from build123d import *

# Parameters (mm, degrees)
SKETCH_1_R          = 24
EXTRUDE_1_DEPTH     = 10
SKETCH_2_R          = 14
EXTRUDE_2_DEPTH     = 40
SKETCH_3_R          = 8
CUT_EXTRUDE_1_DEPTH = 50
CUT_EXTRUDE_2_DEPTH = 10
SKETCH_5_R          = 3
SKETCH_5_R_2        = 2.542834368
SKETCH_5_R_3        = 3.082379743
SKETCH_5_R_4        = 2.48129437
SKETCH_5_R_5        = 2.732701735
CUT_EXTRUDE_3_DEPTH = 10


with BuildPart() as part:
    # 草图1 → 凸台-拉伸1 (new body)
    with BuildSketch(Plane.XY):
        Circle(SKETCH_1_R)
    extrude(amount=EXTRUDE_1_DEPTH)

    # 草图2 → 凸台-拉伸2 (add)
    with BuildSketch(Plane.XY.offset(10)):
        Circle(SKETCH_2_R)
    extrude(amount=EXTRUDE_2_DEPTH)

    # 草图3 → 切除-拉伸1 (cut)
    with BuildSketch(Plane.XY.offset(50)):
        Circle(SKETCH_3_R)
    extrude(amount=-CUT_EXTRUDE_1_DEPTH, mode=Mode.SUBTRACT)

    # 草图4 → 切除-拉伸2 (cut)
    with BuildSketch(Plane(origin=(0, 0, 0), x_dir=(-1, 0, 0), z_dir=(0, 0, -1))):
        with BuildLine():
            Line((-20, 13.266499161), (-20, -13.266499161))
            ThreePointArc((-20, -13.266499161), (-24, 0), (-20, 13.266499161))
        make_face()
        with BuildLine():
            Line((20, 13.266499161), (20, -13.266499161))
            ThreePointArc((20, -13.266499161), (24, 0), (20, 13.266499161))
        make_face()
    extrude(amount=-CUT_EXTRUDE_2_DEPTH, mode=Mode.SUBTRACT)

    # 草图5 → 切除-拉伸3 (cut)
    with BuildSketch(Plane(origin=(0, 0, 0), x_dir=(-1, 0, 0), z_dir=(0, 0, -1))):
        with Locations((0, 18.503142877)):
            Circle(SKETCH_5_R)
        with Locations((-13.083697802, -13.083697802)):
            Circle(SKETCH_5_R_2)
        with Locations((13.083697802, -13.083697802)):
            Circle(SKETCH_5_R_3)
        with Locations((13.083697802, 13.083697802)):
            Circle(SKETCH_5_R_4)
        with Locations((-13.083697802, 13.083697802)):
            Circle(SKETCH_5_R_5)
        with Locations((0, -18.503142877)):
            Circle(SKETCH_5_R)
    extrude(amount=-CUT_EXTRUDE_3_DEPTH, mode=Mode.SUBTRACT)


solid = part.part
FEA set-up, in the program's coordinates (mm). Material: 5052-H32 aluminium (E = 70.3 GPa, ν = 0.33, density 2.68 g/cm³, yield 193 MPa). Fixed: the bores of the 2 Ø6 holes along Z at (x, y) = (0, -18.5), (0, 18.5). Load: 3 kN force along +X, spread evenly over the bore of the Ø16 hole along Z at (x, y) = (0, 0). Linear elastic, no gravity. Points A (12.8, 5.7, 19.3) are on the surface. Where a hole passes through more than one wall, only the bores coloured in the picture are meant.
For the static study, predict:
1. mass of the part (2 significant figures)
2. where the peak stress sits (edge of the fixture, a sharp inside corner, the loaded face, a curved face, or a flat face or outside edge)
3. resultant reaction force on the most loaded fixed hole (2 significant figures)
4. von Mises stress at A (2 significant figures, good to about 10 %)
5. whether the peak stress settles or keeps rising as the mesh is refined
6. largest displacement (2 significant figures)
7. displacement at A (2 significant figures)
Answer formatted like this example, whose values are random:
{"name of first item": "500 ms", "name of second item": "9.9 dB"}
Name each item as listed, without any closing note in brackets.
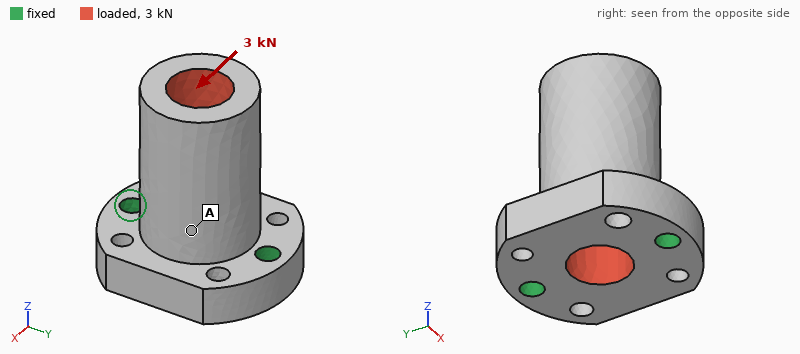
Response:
{"mass of the part": "80 g", "where the peak stress sits": "edge of the fixture", "resultant reaction force on the most loaded fixed hole": "1.5 kN", "von Mises stress at A": "13 MPa", "whether the peak stress settles or keeps rising as the mesh is refined": "keeps rising", "largest displacement": "92 µm", "displacement at A": "35 µm"}
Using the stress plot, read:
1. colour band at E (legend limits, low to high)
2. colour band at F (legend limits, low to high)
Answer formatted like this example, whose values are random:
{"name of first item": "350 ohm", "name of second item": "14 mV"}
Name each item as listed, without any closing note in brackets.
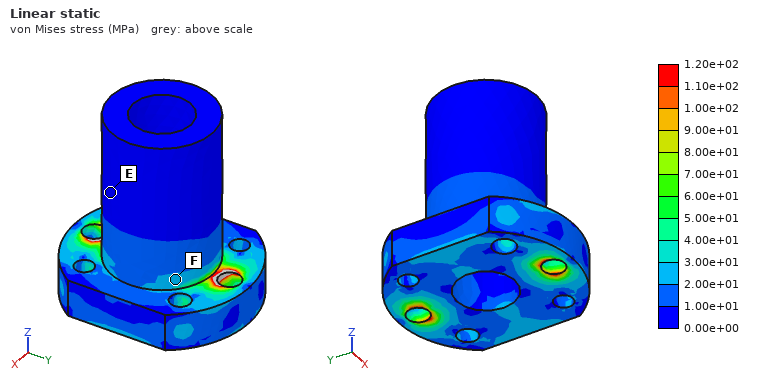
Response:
{"colour band at E": "0.00e+00 to 1.00e+01 MPa", "colour band at F": "2.00e+01 to 3.00e+01 MPa"}
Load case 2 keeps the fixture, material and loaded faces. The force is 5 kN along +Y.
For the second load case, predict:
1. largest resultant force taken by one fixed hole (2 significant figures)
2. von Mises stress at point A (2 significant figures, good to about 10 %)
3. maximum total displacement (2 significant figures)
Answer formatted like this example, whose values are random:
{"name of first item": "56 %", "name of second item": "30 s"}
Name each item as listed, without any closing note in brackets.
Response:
{"largest resultant force taken by one fixed hole": "4.0 kN", "von Mises stress at point A": "18 MPa", "maximum total displacement": "49 µm"}
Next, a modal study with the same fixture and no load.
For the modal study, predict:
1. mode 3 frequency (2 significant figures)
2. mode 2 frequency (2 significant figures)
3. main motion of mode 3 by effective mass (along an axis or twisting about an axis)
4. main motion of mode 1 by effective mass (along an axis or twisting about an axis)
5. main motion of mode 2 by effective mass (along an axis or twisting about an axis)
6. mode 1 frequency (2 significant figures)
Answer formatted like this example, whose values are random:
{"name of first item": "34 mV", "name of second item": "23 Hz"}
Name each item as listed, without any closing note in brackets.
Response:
{"mode 3 frequency": "15 kHz", "mode 2 frequency": "8100 Hz", "main motion of mode 3 by effective mass": "along Z", "main motion of mode 1 by effective mass": "along X", "main motion of mode 2 by effective mass": "along Y", "mode 1 frequency": "4500 Hz"}
